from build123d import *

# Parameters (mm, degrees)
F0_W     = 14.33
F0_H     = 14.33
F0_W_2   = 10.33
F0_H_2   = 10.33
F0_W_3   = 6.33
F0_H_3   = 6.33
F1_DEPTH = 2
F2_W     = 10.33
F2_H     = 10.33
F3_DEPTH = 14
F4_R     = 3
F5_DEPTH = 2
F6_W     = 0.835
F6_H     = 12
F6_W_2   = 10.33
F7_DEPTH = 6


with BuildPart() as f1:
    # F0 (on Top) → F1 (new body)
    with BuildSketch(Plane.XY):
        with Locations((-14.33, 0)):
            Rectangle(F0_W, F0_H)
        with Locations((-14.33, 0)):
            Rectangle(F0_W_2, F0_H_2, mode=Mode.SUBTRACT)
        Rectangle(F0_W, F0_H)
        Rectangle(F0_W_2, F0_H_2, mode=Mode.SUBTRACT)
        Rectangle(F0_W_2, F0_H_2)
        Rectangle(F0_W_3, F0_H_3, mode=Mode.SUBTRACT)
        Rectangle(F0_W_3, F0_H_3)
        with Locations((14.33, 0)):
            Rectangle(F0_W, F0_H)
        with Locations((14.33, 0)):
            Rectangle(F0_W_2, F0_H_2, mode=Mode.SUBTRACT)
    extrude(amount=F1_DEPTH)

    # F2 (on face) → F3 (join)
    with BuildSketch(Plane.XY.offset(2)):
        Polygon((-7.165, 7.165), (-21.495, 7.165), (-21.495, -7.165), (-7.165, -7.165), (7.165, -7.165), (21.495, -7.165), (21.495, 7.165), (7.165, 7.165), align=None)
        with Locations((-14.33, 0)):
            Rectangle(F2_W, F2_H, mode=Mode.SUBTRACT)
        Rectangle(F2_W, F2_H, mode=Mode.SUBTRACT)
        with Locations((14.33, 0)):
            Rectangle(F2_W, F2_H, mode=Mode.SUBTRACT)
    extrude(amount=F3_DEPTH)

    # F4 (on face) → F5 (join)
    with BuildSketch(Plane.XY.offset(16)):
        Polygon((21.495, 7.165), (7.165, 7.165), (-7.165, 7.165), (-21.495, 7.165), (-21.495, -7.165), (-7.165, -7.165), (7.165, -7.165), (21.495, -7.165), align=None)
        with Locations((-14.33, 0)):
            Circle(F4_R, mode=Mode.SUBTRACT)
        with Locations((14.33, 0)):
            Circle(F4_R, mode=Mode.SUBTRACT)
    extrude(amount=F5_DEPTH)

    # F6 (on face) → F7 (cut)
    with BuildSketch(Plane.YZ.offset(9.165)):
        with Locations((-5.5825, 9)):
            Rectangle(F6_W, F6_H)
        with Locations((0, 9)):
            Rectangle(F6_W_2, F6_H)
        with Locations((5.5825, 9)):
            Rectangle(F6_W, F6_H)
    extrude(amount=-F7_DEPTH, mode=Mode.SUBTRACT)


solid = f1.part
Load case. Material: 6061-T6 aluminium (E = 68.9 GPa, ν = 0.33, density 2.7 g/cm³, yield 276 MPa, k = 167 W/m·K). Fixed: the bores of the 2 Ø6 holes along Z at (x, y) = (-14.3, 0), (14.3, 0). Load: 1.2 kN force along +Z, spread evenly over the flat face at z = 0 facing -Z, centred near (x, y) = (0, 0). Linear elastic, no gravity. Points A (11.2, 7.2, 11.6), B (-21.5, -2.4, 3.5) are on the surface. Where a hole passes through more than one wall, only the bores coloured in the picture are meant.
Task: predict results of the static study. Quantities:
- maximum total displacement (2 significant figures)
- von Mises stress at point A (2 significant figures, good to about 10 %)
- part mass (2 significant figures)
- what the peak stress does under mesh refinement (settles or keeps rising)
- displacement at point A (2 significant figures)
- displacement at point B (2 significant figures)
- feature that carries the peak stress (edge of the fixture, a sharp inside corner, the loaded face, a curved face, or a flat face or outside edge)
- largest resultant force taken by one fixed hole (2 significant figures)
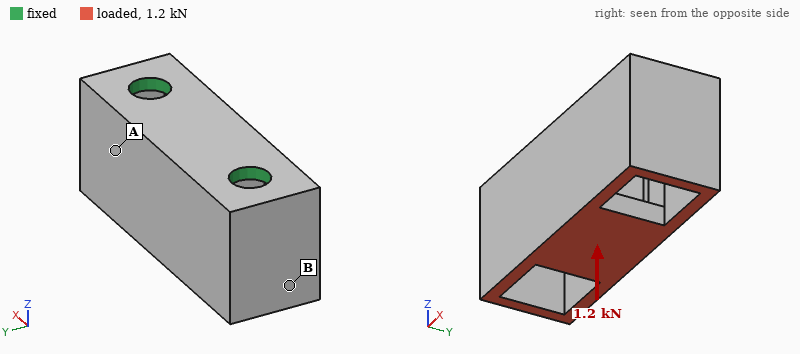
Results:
14 µm
15 MPa
15 g
keeps rising
6.4 µm
3.4 µm
edge of the fixture
650 N
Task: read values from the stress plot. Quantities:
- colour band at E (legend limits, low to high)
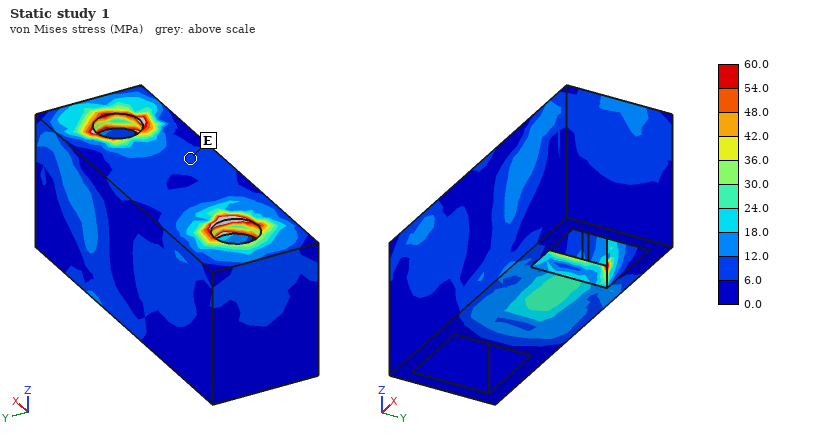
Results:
6.0 to 12.0 MPa
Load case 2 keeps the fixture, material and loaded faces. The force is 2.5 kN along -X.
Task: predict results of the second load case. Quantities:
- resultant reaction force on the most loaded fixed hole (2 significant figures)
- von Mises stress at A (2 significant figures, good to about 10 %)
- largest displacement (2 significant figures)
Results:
1.8 kN
43 MPa
42 µm
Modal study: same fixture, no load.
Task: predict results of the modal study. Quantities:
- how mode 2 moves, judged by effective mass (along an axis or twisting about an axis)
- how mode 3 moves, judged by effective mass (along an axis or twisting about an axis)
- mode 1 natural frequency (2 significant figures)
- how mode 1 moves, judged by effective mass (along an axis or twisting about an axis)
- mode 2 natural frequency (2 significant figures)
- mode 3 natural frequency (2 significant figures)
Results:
twisting about Z
along X
6900 Hz
along Y
16 kHz
17 kHz
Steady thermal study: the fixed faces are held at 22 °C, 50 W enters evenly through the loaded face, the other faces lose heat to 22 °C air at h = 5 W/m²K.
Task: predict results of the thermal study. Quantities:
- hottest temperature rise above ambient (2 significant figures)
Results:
41 K
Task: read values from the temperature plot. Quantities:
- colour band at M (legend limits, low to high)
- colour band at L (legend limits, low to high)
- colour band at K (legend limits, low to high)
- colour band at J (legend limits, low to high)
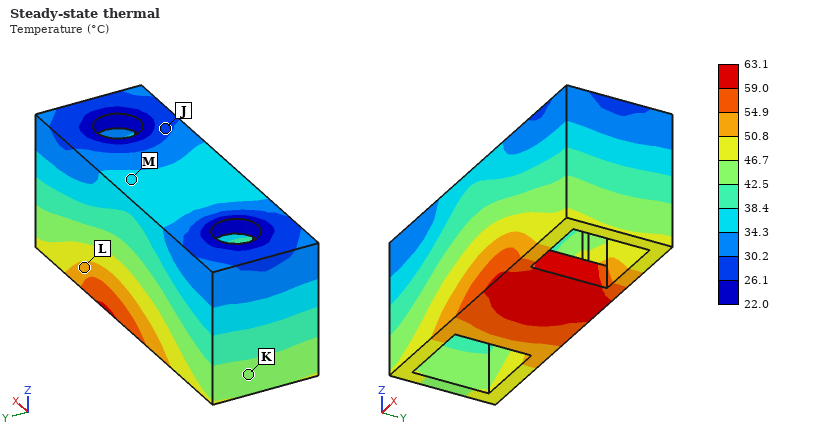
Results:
34.3 to 38.4 °C
50.8 to 54.9 °C
42.5 to 46.7 °C
26.1 to 30.2 °C
